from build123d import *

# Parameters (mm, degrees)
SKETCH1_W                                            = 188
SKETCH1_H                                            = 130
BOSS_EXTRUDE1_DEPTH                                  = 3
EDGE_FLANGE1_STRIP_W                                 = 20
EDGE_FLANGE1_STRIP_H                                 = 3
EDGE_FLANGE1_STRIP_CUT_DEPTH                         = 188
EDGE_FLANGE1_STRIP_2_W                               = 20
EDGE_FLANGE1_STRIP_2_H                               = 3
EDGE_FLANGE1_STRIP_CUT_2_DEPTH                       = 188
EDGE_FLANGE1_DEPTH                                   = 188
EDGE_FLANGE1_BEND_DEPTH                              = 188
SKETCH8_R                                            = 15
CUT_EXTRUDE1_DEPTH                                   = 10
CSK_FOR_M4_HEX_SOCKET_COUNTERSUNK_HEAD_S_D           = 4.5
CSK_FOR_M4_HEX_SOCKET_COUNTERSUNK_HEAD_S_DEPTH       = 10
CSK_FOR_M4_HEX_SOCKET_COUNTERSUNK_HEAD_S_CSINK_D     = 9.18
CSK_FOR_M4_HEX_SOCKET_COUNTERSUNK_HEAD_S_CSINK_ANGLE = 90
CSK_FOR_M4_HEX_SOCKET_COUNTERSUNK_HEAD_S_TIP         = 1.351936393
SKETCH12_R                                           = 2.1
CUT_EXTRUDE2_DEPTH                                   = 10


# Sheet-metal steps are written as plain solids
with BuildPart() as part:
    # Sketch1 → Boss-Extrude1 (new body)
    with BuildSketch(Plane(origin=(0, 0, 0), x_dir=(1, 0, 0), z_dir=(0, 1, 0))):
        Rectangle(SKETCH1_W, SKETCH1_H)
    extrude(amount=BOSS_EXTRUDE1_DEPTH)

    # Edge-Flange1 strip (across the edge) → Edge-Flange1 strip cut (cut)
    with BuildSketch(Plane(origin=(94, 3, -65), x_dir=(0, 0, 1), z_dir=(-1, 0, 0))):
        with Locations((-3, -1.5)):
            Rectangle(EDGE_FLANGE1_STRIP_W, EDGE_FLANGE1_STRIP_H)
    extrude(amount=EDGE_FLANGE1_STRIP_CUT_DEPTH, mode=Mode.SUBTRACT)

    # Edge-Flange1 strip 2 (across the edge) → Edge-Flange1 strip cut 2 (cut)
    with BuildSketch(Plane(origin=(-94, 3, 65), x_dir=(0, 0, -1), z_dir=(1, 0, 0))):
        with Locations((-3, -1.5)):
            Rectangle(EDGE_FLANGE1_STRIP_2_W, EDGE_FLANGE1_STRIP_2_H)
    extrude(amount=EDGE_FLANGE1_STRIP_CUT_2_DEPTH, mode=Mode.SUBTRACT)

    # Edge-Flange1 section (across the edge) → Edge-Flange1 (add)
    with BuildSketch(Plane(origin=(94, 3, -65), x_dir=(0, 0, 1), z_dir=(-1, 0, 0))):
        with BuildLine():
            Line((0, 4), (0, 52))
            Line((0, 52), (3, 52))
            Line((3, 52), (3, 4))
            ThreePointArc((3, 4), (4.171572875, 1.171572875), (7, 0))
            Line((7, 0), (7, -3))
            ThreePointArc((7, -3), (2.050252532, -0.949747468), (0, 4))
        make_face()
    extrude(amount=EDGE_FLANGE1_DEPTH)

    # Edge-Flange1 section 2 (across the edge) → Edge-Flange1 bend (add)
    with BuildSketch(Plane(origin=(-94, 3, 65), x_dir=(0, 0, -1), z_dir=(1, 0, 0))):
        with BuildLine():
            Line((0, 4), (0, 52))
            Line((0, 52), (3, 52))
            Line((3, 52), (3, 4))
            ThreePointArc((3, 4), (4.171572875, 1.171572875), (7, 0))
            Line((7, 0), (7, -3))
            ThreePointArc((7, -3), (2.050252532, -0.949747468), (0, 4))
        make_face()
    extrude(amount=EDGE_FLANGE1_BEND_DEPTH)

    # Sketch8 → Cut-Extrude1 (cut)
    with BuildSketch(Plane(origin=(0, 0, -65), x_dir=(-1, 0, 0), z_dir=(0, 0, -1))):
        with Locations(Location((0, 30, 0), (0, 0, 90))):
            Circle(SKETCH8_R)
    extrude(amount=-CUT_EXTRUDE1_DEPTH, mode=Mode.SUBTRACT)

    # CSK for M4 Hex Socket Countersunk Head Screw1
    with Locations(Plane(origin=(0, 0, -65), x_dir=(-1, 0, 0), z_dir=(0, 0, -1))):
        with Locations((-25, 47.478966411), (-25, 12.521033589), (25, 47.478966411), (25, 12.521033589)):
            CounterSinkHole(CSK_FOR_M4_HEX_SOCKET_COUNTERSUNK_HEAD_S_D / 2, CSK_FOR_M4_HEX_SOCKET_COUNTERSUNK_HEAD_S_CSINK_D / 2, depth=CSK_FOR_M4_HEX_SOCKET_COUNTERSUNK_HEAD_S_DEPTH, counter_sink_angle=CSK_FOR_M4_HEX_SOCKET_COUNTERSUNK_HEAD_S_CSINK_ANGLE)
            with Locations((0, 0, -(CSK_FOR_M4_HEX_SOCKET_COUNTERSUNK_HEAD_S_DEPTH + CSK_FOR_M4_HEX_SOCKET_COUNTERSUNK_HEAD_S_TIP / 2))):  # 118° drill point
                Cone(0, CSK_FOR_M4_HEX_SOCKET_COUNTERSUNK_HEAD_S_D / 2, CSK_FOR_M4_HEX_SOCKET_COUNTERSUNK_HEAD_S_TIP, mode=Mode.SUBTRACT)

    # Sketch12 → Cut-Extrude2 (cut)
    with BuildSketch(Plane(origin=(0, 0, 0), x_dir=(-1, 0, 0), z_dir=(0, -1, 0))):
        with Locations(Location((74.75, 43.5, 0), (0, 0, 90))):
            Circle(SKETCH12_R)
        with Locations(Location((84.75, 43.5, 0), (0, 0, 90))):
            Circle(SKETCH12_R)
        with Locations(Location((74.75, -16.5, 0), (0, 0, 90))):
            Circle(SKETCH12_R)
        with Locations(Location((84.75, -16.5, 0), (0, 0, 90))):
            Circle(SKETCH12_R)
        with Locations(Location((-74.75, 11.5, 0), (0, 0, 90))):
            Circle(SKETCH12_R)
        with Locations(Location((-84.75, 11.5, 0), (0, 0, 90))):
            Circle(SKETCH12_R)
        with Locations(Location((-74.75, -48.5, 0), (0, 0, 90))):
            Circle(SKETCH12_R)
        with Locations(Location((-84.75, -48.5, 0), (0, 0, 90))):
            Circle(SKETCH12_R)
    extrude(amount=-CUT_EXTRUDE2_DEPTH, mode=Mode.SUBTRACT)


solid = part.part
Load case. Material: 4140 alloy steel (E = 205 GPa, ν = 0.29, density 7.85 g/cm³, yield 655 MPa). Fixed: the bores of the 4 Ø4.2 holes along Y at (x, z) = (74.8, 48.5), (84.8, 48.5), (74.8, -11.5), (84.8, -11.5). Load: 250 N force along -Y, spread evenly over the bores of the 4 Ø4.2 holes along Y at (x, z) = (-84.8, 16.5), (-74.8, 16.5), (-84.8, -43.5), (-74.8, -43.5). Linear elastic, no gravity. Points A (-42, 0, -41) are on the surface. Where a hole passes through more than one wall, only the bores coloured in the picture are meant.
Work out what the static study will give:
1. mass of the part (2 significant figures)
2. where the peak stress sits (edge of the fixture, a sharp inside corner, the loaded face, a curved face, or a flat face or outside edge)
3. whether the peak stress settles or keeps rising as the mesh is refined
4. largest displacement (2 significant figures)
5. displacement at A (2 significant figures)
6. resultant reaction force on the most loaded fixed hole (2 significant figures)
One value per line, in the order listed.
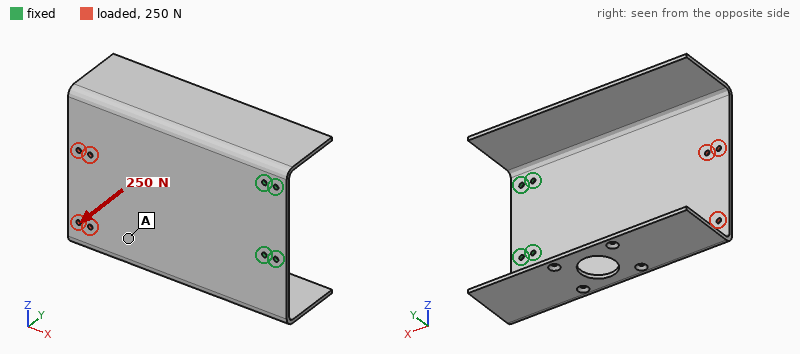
990 g
edge of the fixture
keeps rising
2.4 mm
1.4 mm
1.3 kN
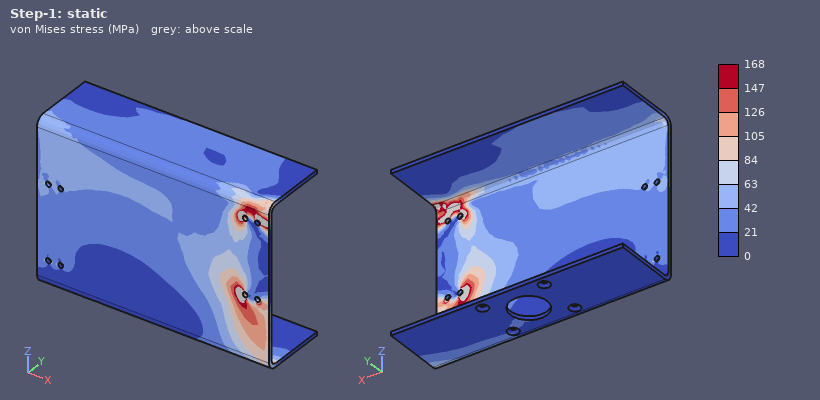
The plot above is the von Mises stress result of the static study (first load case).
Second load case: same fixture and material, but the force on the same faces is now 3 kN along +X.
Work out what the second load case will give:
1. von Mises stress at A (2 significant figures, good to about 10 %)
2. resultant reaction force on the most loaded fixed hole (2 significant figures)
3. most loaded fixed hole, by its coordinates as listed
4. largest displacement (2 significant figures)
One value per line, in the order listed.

11 MPa
2.0 kN
(74.8, -11.5)
24 µm
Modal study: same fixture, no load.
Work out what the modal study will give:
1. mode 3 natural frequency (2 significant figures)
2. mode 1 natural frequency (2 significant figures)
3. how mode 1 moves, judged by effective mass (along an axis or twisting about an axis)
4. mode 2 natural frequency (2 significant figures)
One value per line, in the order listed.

340 Hz
110 Hz
along Y
180 Hz
